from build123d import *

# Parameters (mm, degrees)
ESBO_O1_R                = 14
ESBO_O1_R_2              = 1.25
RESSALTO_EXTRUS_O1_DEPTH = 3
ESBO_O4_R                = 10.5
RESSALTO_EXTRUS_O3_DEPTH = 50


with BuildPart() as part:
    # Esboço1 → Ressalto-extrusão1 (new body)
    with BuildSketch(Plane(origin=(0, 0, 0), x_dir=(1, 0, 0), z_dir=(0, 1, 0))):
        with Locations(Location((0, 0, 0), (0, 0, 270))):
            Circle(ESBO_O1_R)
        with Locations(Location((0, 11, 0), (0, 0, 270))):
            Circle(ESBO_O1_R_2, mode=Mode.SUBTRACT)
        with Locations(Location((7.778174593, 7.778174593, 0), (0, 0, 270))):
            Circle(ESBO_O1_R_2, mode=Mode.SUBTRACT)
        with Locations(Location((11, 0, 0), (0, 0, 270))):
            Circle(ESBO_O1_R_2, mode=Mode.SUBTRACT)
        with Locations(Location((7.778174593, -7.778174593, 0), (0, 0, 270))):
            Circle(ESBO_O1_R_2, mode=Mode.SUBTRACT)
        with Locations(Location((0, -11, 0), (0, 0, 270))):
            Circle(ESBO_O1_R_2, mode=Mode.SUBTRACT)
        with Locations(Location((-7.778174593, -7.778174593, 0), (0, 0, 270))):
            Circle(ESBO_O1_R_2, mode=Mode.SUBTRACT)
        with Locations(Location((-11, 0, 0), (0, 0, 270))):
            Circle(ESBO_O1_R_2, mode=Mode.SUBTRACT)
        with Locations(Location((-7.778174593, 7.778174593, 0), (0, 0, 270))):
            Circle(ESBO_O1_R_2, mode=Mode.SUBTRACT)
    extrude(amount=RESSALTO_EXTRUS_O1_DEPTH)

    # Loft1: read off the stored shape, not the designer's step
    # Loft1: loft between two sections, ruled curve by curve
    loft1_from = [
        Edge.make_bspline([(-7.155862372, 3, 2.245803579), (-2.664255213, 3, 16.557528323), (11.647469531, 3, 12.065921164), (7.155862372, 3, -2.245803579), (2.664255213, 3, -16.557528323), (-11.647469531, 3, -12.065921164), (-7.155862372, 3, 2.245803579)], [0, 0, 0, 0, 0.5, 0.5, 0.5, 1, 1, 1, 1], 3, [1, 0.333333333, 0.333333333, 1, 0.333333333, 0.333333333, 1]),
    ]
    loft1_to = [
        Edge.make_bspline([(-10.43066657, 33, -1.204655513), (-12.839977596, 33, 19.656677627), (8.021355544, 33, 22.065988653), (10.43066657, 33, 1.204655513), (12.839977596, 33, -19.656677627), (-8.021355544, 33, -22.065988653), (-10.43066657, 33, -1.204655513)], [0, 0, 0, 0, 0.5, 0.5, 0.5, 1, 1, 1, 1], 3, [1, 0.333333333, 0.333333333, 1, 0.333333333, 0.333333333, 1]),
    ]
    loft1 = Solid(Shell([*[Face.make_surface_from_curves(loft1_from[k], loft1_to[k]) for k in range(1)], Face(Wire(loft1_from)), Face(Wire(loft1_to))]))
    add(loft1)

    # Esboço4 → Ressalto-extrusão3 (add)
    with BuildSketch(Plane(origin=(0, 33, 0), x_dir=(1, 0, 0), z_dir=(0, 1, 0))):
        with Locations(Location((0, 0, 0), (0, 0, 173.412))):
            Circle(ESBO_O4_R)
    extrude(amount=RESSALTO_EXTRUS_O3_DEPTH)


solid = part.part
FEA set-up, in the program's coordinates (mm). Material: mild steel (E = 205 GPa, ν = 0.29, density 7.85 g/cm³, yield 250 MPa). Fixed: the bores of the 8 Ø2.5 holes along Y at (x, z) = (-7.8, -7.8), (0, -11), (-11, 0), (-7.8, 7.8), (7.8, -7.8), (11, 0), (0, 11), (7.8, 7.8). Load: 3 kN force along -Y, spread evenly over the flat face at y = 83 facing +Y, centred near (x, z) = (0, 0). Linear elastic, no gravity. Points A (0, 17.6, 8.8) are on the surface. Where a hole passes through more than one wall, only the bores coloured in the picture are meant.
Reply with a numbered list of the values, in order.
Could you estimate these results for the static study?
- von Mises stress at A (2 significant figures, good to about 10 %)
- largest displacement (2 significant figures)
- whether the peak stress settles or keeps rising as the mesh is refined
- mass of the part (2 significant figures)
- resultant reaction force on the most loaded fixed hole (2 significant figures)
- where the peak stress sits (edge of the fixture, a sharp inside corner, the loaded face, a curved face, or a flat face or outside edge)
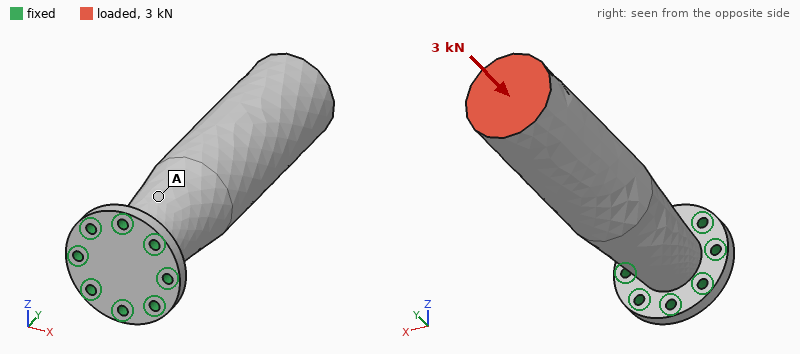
1. 12 MPa
2. 6.0 µm
3. keeps rising
4. 210 g
5. 410 N
6. edge of the fixture
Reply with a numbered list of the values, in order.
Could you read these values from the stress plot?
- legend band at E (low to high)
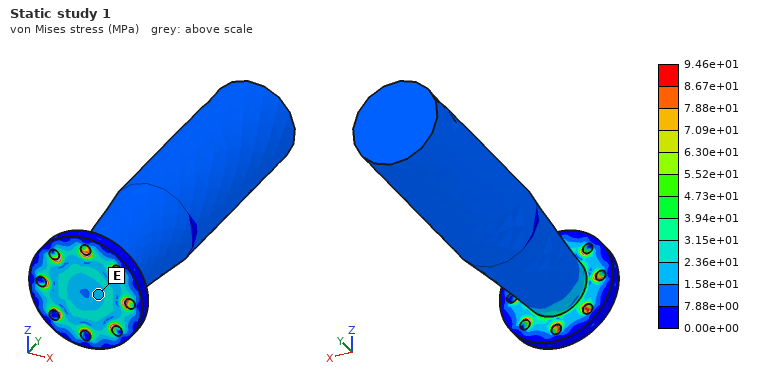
1. 1.58e+01 to 2.36e+01 MPa
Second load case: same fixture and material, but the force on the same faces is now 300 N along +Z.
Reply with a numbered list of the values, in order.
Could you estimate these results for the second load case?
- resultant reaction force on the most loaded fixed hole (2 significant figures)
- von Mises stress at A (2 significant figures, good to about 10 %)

1. 680 N
2. 37 MPa
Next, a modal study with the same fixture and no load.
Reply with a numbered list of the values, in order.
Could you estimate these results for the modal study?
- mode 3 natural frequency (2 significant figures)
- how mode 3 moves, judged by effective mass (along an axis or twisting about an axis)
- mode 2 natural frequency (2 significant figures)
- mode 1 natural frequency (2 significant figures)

1. 7000 Hz
2. twisting about Y
3. 1200 Hz
4. 1200 Hz
